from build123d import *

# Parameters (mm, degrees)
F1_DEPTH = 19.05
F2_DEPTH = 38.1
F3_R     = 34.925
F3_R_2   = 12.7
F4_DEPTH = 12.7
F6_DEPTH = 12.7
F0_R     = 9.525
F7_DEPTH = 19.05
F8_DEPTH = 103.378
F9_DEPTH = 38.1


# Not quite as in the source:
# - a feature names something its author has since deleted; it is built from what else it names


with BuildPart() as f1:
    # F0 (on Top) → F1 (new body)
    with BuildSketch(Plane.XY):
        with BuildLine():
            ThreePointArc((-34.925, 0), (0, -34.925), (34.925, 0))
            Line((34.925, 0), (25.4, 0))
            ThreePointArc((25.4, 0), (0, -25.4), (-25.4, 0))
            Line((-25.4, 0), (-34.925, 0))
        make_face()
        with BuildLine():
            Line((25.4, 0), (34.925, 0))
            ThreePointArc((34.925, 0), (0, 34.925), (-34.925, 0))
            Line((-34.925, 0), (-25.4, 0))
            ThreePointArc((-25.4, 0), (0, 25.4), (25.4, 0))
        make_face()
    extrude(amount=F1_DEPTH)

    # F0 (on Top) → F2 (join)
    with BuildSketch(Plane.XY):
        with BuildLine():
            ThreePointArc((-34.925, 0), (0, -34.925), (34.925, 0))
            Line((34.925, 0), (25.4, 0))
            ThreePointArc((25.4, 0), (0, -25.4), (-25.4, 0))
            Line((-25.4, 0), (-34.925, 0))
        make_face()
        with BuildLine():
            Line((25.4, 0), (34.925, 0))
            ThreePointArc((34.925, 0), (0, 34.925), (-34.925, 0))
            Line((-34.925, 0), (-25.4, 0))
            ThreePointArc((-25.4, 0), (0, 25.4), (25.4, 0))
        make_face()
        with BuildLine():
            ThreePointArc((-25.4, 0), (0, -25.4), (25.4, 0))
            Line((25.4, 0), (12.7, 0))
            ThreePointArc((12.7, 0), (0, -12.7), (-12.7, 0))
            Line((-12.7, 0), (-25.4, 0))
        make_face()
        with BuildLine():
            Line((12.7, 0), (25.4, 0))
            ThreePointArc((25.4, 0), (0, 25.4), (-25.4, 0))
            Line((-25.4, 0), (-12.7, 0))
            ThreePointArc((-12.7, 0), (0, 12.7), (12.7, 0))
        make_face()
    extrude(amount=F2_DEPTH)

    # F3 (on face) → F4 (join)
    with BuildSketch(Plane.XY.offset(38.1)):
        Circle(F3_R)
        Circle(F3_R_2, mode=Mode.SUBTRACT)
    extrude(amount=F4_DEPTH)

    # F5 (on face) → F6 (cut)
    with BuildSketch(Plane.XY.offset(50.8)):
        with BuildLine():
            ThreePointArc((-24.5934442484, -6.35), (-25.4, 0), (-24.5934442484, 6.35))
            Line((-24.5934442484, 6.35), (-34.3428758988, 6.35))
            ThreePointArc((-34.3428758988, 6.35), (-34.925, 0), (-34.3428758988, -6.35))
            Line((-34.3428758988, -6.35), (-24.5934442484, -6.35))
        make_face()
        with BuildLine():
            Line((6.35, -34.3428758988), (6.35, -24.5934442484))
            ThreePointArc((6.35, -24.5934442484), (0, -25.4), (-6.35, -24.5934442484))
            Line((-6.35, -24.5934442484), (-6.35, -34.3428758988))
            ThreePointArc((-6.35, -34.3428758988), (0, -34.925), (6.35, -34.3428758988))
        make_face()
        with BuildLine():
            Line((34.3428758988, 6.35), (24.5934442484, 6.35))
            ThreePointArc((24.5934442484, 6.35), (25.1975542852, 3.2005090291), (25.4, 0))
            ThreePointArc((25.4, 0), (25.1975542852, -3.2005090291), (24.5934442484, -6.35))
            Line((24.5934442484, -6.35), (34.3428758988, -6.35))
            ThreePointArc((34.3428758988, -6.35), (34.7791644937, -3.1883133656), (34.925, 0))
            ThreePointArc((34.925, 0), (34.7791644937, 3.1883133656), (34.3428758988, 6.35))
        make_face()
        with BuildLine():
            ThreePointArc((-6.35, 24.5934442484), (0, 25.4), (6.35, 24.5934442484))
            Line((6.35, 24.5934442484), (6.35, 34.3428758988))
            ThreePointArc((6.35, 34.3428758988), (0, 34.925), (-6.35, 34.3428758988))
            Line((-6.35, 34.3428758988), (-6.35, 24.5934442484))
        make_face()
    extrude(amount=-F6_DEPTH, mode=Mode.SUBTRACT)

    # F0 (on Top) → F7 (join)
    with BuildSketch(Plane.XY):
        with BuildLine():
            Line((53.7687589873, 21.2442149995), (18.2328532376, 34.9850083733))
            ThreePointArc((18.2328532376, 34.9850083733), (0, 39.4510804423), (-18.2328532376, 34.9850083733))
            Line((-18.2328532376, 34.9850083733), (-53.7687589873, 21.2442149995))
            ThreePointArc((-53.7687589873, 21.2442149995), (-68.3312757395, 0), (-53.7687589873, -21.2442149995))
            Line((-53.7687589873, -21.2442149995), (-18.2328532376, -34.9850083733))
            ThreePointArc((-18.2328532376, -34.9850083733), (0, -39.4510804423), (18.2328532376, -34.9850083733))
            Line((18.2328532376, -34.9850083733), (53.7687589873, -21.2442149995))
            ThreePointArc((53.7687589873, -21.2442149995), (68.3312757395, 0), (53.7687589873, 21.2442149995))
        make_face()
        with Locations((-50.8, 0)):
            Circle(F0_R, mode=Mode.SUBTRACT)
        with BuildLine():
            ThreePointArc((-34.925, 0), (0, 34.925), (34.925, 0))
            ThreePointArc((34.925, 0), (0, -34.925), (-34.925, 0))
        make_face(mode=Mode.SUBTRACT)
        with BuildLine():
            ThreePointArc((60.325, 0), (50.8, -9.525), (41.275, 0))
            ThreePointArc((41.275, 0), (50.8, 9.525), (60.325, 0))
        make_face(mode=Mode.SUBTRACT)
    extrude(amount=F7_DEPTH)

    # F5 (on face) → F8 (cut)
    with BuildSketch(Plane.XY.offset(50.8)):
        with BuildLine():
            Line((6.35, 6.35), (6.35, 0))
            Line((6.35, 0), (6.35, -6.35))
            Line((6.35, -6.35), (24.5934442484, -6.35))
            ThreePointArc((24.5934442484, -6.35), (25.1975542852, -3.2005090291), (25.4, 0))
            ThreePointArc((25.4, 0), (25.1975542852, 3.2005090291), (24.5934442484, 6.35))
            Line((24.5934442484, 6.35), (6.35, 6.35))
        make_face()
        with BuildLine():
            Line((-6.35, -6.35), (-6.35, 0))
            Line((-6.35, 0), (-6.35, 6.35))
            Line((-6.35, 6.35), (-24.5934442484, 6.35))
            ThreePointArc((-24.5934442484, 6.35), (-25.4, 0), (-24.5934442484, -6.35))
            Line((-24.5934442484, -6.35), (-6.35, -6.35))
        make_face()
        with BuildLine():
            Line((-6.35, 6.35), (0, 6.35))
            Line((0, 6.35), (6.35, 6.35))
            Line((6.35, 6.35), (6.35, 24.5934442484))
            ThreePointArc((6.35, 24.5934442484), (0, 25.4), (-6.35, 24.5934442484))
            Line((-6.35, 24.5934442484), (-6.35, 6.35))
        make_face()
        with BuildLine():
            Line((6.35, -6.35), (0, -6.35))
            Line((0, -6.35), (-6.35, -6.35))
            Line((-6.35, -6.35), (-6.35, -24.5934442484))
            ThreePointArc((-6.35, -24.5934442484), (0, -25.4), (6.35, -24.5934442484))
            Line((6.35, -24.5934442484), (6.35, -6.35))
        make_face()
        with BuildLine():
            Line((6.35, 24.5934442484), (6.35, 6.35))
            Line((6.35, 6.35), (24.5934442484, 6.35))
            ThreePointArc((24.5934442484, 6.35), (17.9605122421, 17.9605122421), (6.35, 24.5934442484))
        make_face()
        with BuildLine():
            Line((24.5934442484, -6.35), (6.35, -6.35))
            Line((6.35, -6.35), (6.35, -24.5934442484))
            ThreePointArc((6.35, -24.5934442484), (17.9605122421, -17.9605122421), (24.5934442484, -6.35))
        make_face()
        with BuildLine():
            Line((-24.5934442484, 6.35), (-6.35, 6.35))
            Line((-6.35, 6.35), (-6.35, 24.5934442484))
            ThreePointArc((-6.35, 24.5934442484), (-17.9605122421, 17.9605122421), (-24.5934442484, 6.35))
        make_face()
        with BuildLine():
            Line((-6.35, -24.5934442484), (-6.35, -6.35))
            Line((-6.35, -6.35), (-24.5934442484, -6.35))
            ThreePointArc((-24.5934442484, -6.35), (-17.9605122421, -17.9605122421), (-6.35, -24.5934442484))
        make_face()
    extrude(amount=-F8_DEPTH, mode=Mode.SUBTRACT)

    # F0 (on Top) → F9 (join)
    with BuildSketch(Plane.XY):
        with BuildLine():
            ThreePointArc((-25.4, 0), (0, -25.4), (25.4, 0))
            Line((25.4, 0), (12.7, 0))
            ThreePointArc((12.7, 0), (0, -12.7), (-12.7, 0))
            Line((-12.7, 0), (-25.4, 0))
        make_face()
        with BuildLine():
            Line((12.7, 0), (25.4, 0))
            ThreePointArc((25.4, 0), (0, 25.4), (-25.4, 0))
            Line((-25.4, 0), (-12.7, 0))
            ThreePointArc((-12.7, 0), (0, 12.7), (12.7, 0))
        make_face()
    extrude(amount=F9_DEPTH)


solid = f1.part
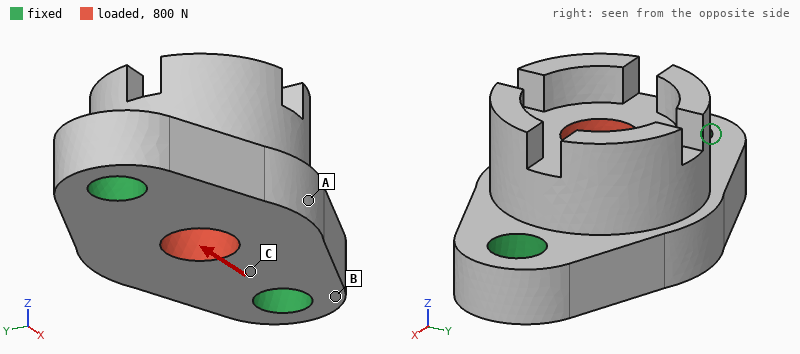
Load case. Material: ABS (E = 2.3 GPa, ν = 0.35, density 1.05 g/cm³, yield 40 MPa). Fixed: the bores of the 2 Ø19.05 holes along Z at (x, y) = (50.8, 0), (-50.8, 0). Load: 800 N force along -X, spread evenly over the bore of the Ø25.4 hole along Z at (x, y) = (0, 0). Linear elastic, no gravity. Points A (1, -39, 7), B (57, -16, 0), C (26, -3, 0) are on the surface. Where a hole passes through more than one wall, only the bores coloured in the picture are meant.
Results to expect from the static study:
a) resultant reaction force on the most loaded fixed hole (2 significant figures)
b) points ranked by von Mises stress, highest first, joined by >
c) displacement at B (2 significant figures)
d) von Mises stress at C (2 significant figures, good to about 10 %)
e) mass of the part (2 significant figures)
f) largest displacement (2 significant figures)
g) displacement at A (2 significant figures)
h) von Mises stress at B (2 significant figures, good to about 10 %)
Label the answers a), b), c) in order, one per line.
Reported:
a) 410 N
b) C > B > A
c) 1.7 µm
d) 0.36 MPa
e) 220 g
f) 11 µm
g) 3.9 µm
h) 0.23 MPa
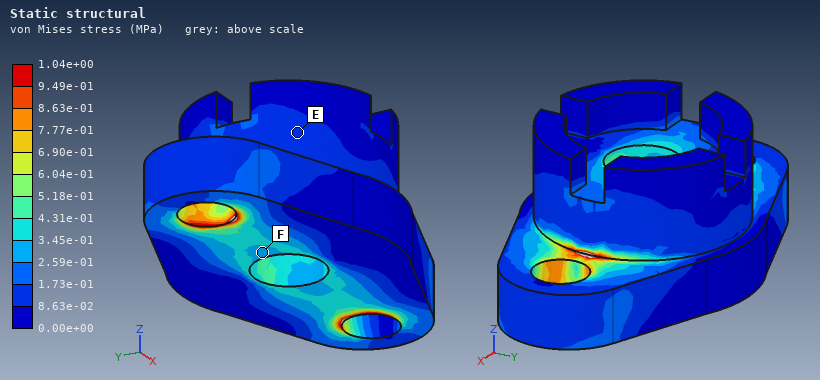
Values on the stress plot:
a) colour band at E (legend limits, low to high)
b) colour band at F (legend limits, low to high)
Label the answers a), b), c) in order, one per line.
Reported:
a) 8.63e-02 to 1.73e-01 MPa
b) 2.59e-01 to 3.45e-01 MPa
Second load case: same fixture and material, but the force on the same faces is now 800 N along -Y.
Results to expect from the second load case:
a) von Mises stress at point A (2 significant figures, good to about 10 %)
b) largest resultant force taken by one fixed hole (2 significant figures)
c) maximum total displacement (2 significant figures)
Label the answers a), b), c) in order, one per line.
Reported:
a) 0.41 MPa
b) 400 N
c) 55 µm
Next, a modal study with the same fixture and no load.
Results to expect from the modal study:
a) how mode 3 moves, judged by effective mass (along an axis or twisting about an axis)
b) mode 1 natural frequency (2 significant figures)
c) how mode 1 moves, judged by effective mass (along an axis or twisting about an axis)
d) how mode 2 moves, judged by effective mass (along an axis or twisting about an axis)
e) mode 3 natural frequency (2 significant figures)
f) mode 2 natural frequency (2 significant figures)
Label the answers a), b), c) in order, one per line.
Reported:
a) along Y
b) 1400 Hz
c) along Y
d) along Z
e) 3300 Hz
f) 2200 Hz
